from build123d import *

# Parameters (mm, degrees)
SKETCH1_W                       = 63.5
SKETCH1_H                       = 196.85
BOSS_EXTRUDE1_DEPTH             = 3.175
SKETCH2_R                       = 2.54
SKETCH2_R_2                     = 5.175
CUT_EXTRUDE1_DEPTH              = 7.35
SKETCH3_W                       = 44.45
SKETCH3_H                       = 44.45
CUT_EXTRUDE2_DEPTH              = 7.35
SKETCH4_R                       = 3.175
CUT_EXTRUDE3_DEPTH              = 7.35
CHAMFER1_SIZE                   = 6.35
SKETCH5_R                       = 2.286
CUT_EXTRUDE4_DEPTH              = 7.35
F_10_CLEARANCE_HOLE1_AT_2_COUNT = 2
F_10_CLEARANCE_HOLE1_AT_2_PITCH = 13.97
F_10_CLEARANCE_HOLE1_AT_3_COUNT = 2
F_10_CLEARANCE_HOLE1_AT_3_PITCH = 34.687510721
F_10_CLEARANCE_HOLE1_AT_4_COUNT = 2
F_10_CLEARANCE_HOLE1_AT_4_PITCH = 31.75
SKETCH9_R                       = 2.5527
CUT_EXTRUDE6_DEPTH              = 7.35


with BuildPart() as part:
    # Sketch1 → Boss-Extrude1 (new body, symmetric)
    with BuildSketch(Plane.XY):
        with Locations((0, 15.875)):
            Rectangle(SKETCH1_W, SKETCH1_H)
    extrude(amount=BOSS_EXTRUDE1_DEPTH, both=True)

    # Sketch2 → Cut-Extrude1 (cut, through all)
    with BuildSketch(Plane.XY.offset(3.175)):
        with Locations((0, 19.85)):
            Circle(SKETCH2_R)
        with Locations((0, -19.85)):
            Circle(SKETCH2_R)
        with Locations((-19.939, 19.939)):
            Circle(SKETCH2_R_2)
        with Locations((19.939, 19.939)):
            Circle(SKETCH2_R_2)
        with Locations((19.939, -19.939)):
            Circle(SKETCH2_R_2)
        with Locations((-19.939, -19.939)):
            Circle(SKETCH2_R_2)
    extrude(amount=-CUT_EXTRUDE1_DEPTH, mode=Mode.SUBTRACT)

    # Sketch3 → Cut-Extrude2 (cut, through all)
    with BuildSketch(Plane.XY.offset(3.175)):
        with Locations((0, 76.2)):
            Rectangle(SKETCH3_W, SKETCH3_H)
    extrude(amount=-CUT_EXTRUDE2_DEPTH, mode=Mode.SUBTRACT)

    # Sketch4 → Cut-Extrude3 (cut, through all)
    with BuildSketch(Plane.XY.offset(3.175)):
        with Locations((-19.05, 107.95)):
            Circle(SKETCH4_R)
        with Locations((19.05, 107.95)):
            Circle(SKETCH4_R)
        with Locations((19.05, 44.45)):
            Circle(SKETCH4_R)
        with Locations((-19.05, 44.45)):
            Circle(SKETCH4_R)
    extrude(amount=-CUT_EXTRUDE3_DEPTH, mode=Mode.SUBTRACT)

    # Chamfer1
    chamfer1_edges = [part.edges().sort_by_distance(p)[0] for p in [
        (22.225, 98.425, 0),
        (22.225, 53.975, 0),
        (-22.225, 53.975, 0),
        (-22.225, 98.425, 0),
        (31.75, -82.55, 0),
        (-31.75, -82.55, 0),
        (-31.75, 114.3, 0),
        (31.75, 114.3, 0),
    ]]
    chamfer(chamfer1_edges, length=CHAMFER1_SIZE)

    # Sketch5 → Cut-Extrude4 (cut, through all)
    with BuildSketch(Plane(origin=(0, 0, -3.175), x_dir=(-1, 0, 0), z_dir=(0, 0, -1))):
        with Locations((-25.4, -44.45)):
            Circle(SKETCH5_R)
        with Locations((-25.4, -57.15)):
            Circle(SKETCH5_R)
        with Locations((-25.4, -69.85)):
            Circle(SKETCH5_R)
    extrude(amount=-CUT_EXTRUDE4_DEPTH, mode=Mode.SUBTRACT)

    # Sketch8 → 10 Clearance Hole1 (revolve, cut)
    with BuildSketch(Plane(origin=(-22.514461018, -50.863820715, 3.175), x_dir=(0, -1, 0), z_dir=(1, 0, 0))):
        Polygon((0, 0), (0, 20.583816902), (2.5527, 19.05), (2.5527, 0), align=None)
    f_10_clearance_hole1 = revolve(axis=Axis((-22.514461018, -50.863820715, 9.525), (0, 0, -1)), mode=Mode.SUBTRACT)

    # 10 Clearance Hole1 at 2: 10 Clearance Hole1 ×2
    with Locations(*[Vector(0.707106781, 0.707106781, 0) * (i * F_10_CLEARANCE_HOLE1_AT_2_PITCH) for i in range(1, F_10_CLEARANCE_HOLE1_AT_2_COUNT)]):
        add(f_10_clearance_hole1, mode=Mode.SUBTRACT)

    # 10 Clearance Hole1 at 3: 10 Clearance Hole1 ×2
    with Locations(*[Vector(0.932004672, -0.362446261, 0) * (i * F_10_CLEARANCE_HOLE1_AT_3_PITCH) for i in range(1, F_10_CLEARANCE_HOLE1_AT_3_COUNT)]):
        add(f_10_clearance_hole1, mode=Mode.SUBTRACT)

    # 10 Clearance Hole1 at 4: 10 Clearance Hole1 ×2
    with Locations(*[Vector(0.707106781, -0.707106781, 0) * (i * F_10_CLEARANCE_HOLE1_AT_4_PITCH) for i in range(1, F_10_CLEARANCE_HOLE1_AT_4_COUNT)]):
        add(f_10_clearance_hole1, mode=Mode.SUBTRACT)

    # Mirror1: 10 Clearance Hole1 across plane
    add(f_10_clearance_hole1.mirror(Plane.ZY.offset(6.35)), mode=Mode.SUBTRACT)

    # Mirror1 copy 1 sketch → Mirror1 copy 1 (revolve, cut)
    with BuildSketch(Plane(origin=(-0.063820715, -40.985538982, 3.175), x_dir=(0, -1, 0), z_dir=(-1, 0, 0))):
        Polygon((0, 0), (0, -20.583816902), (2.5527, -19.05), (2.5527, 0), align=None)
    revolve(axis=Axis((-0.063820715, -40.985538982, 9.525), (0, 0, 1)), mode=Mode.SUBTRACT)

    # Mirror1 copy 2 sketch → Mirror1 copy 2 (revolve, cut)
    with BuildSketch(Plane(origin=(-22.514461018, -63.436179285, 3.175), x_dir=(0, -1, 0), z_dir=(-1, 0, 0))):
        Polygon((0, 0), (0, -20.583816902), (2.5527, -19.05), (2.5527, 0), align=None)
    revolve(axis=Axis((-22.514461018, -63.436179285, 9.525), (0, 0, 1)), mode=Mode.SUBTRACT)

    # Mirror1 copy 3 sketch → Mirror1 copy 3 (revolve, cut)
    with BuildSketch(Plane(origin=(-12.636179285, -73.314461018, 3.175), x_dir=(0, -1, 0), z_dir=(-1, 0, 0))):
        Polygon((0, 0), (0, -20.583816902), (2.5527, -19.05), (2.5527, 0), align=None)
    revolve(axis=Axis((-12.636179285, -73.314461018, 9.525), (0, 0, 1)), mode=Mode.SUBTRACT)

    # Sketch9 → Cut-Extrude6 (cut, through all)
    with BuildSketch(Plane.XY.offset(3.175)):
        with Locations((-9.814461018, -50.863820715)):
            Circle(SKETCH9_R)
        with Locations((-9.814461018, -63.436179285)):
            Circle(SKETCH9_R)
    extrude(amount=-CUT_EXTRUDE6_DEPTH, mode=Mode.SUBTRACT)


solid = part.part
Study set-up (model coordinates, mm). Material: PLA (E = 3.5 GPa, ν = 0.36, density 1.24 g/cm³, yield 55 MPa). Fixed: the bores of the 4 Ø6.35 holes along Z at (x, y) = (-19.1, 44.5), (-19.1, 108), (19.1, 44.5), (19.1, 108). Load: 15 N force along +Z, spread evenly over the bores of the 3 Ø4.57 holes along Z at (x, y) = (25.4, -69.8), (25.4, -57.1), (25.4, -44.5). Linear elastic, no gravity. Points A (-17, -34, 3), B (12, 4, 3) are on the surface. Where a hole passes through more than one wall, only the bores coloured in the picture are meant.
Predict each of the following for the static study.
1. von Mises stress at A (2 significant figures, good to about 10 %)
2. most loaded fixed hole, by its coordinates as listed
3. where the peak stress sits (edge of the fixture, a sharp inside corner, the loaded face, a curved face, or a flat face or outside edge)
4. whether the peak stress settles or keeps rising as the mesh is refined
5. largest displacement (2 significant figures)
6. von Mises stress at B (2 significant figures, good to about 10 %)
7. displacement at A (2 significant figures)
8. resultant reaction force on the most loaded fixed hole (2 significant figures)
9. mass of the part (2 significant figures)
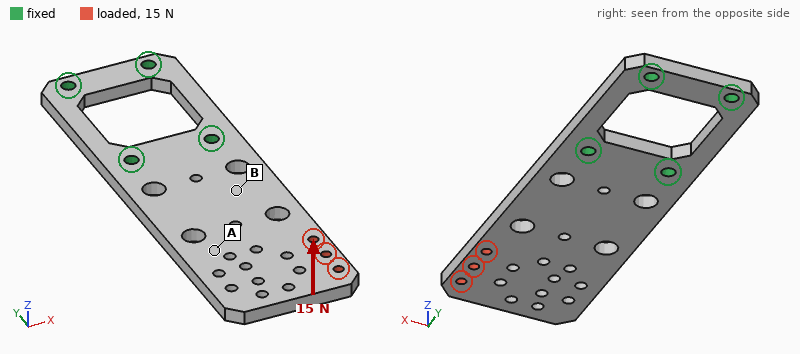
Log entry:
0.89 MPa
(19.1, 44.5)
edge of the fixture
keeps rising
1.9 mm
2.3 MPa
0.77 mm
17 N
77 g
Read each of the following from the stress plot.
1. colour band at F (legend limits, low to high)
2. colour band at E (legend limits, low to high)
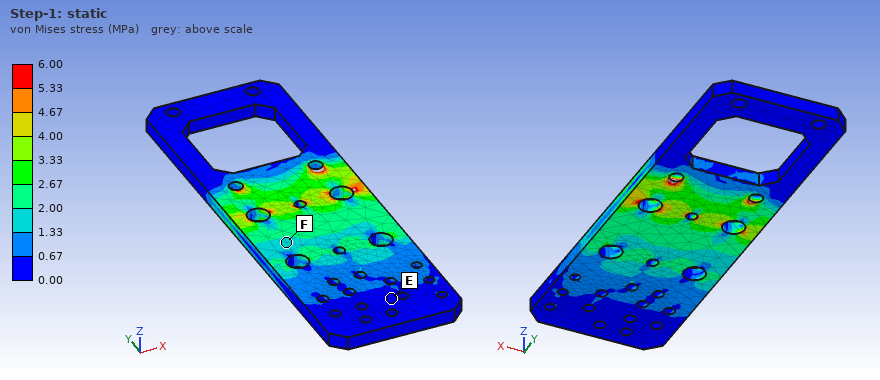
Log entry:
1.33 to 2.00 MPa
0.00 to 0.67 MPa
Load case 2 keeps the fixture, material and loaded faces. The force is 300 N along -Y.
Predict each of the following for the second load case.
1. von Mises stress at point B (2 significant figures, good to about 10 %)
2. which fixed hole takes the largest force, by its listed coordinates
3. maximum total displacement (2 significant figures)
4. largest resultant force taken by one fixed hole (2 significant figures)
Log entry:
1.4 MPa
(19.1, 44.5)
0.19 mm
310 N
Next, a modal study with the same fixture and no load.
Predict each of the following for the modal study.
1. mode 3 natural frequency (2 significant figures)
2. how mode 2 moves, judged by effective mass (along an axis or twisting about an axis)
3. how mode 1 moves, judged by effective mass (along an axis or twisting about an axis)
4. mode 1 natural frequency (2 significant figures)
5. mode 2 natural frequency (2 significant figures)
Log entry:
650 Hz
twisting about Y
along Z
110 Hz
440 Hz
